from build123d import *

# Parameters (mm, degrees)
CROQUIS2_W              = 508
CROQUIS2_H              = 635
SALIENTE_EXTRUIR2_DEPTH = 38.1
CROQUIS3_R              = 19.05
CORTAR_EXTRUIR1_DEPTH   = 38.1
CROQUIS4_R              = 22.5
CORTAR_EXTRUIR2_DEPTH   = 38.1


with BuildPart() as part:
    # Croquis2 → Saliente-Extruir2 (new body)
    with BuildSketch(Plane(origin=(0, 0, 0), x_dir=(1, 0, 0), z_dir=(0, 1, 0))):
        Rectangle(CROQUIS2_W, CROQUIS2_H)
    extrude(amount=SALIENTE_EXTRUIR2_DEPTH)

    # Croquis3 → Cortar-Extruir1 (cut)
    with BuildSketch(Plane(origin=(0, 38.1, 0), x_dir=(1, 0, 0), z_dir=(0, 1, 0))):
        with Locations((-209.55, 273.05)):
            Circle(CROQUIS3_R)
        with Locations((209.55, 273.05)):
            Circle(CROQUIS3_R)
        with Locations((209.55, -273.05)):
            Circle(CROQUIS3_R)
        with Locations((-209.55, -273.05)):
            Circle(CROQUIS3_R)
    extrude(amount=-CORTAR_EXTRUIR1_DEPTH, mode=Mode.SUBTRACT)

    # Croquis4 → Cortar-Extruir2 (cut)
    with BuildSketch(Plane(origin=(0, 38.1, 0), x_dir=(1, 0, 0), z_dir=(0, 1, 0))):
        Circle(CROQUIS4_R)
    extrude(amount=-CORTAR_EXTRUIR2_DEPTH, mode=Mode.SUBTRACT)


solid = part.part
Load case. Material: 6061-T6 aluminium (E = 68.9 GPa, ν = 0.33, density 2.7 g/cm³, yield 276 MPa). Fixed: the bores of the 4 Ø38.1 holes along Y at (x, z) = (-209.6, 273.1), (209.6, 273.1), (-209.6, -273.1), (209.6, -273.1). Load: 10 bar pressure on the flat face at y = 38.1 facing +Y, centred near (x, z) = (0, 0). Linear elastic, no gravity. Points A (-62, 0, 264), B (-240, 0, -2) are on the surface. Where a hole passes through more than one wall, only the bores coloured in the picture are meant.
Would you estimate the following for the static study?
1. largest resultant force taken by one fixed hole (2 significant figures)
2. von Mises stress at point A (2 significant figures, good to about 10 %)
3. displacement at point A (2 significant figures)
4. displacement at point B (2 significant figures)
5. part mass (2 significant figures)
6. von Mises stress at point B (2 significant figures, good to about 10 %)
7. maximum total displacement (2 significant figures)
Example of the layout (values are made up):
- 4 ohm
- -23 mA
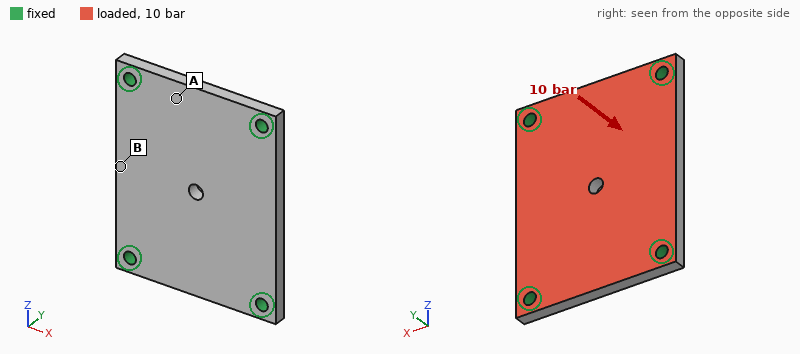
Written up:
- 79 kN
- 31 MPa
- 0.35 mm
- 0.94 mm
- 33 kg
- 67 MPa
- 1.3 mm
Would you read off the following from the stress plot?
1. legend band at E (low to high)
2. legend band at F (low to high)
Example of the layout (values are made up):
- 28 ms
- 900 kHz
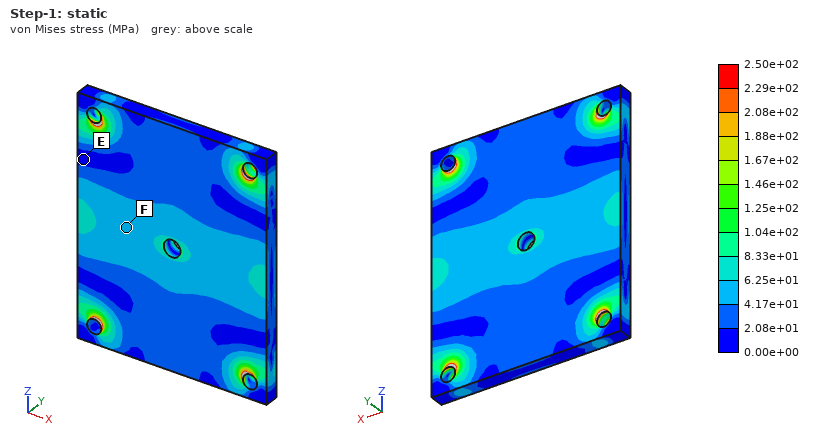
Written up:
- 0.00e+00 to 2.08e+01 MPa
- 4.17e+01 to 6.25e+01 MPa
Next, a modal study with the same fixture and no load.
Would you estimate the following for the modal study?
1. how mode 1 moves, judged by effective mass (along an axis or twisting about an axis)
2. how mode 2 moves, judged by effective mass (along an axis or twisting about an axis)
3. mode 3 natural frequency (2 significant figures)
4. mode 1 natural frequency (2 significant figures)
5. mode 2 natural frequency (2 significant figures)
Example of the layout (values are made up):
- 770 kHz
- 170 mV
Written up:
- along Y
- twisting about Z
- 1100 Hz
- 530 Hz
- 800 Hz
